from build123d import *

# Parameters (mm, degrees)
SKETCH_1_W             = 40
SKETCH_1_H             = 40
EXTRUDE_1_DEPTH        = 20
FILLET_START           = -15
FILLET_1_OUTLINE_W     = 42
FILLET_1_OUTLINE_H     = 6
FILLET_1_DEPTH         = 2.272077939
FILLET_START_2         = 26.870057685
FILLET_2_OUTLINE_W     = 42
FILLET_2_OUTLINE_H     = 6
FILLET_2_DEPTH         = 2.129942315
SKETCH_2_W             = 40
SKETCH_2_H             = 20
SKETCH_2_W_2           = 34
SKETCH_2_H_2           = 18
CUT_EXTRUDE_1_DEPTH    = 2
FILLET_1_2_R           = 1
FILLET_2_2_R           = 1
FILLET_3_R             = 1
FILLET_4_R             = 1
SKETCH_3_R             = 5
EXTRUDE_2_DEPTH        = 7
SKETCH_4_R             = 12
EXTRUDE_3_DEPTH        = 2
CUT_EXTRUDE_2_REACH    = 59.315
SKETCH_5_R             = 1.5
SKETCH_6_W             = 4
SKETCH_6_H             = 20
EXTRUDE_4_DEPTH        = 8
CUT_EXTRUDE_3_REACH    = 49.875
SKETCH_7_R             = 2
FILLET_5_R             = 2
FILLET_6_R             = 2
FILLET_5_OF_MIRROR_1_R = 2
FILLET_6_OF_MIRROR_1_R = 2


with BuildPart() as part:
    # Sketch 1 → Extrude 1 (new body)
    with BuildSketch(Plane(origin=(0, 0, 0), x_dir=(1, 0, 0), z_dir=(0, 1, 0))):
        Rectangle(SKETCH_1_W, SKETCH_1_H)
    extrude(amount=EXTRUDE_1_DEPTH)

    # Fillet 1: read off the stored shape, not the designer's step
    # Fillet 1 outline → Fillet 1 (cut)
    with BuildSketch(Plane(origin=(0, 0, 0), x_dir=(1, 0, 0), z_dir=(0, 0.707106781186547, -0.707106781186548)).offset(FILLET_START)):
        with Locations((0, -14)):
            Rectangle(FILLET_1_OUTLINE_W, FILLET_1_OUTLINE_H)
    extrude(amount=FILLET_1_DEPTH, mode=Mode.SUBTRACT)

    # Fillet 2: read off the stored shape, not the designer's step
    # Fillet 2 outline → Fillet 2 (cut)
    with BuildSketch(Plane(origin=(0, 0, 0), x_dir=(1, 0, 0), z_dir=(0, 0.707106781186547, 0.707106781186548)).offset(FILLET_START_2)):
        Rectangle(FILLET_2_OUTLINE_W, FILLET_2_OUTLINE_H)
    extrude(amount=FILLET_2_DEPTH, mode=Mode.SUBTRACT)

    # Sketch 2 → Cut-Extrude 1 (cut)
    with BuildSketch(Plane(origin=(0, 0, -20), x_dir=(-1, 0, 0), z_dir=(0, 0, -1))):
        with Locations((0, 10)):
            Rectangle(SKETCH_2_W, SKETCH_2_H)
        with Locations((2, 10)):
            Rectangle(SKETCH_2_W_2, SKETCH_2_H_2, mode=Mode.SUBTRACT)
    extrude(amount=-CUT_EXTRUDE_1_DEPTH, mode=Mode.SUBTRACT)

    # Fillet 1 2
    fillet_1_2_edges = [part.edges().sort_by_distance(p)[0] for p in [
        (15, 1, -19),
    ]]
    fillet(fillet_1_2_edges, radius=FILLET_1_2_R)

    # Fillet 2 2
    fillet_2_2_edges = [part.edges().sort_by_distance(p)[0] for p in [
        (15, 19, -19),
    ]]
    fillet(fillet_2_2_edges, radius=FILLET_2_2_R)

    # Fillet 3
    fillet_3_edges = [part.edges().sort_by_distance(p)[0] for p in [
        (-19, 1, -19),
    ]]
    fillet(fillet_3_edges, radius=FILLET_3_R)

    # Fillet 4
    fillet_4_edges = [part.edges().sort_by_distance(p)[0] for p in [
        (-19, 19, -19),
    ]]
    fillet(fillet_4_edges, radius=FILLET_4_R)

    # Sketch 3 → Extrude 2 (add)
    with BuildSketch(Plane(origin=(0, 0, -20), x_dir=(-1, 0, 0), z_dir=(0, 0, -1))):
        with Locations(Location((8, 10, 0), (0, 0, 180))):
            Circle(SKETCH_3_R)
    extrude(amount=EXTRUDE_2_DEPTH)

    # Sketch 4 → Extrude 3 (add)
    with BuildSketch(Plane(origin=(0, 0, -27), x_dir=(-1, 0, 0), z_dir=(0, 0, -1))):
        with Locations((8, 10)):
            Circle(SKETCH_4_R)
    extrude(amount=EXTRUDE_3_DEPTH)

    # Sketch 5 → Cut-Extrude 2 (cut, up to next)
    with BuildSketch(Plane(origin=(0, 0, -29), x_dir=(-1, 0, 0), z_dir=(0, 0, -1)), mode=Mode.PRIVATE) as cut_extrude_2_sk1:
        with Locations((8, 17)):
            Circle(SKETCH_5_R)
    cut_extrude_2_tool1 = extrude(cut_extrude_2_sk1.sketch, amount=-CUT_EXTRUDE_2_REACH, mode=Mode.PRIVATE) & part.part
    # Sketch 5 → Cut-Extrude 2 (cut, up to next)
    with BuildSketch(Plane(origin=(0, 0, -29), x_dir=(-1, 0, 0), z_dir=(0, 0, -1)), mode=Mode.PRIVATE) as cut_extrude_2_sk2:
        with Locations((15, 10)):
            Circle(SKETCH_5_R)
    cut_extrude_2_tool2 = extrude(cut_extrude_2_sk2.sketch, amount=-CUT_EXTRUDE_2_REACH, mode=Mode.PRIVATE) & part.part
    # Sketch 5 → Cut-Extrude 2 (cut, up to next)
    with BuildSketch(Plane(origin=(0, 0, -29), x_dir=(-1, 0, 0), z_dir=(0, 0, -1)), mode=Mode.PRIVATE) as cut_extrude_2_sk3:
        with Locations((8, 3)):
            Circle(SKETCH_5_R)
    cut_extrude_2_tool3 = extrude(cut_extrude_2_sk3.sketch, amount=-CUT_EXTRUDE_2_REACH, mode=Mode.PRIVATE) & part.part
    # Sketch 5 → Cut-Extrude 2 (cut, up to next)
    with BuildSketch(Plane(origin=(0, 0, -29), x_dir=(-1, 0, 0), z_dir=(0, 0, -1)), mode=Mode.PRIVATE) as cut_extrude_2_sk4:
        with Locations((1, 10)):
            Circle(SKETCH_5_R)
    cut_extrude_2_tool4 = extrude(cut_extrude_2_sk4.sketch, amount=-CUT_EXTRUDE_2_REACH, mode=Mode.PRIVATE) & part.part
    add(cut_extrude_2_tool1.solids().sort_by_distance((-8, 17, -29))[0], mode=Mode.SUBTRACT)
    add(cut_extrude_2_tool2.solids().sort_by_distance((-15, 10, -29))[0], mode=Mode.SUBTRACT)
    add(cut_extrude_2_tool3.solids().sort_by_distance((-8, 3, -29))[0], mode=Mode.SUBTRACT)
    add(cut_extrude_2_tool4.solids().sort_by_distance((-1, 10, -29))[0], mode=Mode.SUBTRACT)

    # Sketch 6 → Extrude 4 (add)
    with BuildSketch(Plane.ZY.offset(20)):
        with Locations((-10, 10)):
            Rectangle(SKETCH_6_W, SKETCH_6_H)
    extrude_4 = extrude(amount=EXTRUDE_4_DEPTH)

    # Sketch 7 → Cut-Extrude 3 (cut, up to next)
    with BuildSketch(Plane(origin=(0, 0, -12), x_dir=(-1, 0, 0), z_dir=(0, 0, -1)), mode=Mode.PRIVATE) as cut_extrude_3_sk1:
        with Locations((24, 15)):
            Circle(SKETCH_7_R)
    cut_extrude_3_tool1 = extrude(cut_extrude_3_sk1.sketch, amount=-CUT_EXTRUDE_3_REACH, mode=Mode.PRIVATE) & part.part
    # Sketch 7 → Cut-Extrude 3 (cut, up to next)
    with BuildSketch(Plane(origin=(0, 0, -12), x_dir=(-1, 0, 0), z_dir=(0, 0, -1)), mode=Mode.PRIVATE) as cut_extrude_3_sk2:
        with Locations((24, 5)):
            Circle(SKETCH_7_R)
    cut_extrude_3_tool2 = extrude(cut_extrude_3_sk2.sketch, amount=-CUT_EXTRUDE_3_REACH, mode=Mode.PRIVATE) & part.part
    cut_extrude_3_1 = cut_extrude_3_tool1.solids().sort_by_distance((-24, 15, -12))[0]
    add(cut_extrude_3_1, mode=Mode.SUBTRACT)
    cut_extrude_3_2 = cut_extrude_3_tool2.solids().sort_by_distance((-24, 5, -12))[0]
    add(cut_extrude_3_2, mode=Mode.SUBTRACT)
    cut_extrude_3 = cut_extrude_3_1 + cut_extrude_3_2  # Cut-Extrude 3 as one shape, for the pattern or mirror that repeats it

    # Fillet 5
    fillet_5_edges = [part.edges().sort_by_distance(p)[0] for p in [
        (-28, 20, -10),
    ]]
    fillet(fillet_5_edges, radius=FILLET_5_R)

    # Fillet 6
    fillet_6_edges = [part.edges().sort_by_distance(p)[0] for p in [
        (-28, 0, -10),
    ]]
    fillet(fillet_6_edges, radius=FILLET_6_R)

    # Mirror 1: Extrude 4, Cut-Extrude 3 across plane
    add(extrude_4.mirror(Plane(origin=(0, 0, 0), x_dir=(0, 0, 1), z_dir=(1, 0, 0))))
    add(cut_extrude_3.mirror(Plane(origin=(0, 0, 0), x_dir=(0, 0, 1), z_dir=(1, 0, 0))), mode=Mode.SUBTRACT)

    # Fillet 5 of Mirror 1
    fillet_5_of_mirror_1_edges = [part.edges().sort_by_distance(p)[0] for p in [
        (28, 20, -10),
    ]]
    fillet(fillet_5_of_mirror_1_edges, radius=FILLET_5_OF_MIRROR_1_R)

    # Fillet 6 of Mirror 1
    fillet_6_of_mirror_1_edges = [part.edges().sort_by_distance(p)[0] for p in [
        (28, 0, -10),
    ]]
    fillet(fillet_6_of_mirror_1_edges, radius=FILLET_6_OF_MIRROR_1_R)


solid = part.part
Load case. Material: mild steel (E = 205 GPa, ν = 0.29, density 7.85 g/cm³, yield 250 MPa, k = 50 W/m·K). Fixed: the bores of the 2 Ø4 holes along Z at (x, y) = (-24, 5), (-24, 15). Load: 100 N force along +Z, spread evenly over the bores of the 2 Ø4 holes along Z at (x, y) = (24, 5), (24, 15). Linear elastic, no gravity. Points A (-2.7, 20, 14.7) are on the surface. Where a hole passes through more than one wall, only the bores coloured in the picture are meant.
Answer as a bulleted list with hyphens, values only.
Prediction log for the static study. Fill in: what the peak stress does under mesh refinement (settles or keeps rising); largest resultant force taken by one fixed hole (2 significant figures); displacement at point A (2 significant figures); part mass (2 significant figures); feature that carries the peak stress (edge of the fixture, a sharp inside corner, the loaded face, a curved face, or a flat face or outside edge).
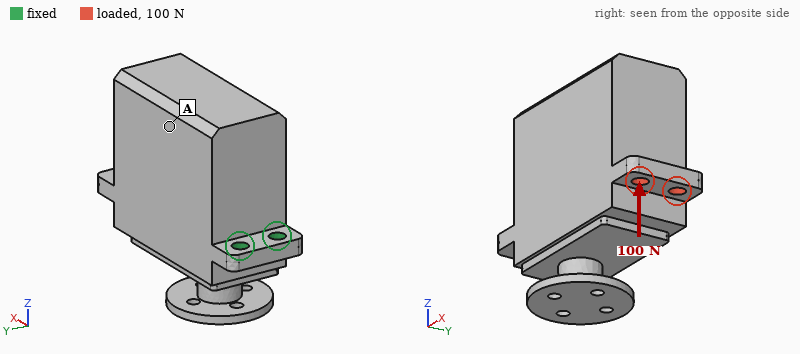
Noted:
- keeps rising
- 50 N
- 27 µm
- 270 g
- edge of the fixture
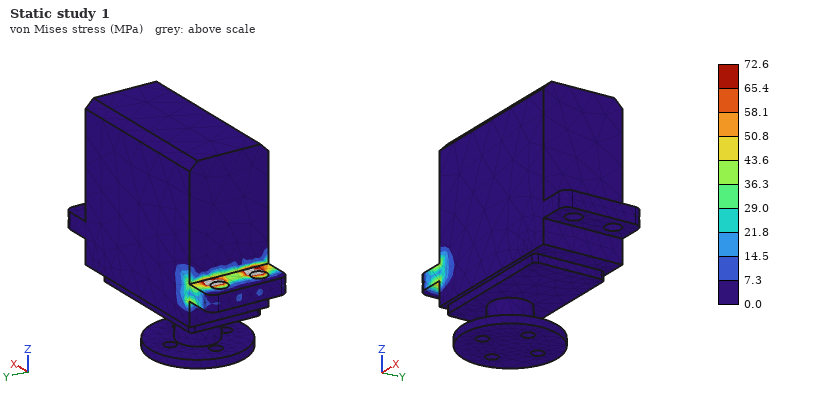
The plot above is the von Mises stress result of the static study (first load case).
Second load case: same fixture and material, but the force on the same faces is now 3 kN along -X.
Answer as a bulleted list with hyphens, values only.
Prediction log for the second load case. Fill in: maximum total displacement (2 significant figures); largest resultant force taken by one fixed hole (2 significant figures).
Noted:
- 5.4 µm
- 1.5 kN
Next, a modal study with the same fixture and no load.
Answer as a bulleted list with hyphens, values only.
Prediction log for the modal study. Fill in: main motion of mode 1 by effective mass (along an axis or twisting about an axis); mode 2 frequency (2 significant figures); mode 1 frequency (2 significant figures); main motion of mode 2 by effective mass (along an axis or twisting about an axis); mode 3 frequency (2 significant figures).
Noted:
- along Z
- 2600 Hz
- 780 Hz
- along Y
- 4300 Hz
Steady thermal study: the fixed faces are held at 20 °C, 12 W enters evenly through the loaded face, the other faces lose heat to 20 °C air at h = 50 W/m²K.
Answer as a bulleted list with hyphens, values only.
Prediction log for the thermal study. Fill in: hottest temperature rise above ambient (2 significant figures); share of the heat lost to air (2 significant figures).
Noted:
- 45 K
- 45 %
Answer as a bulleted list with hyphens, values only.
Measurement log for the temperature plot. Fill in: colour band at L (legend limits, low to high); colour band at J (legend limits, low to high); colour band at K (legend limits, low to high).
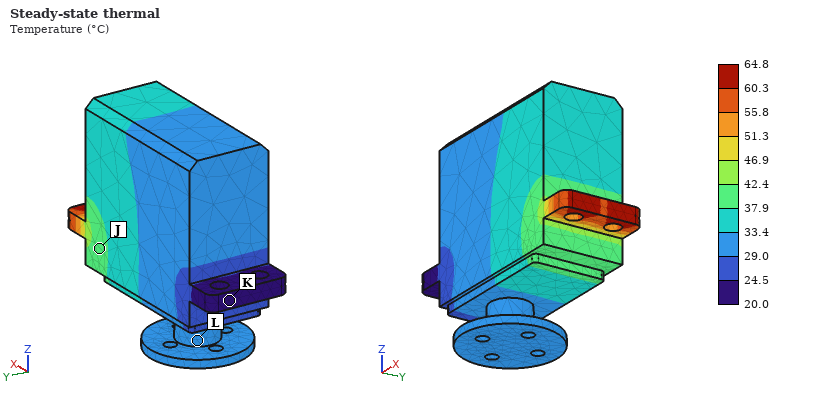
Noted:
- 29.0 to 33.4 °C
- 37.9 to 42.4 °C
- 20.0 to 24.5 °C
